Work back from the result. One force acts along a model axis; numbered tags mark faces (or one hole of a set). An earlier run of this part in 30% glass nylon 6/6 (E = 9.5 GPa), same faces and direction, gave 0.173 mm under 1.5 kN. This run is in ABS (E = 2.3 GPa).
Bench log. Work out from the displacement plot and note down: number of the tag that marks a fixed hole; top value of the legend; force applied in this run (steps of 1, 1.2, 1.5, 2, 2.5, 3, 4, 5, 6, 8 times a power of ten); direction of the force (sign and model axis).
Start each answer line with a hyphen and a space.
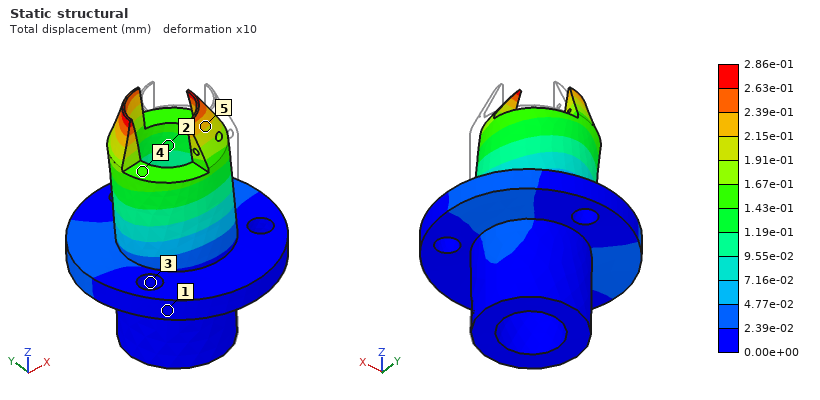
- 3
- 2.86e-01 mm
- 600 N
- -X
